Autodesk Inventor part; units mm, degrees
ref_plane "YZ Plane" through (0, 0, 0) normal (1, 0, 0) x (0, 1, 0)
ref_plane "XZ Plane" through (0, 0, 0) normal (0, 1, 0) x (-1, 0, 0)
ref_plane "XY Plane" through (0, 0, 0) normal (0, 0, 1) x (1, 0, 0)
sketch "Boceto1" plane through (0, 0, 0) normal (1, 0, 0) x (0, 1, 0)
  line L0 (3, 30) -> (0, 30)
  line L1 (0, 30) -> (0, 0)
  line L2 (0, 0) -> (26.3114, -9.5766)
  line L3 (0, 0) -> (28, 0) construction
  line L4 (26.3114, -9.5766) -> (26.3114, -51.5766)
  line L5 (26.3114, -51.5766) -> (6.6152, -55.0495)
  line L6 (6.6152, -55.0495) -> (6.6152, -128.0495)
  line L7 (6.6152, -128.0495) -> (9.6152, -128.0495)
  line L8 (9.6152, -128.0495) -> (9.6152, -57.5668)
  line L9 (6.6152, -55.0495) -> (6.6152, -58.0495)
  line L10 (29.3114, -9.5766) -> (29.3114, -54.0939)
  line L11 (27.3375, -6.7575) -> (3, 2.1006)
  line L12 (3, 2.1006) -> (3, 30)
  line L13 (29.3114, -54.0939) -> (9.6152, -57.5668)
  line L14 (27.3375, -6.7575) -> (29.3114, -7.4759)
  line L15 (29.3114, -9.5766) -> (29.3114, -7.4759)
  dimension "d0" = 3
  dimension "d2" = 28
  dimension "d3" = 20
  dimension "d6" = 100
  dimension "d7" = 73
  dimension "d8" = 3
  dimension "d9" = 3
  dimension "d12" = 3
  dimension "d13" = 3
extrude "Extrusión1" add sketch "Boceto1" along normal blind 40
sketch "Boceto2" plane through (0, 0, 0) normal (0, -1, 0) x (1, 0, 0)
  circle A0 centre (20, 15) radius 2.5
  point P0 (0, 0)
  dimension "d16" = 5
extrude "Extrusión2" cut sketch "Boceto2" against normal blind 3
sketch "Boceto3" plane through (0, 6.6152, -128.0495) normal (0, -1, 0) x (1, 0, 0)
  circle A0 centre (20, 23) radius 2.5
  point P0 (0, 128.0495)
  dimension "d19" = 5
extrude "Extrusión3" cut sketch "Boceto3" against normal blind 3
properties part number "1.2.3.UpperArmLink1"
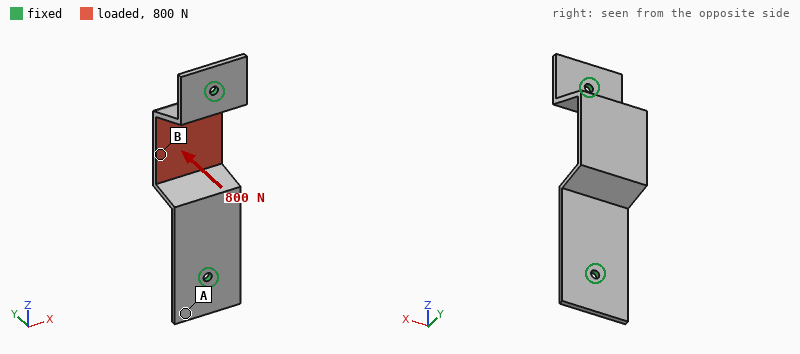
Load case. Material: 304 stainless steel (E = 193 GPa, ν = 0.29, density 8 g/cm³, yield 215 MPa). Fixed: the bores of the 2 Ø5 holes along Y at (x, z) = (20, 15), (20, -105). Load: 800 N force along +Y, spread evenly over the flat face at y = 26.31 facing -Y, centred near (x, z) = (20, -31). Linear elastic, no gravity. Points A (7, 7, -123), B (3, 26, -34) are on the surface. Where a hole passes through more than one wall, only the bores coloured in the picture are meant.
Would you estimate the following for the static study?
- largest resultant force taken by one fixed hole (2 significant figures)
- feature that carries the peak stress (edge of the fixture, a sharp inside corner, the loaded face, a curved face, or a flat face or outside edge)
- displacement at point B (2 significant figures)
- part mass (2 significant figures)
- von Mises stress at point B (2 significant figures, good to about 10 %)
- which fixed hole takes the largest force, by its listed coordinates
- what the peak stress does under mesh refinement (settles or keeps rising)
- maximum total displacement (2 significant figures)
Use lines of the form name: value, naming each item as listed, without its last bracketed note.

largest resultant force taken by one fixed hole: 680 N
feature that carries the peak stress: edge of the fixture
displacement at point B: 0.14 mm
part mass: 180 g
von Mises stress at point B: 28 MPa
which fixed hole takes the largest force, by its listed coordinates: (20, 15)
what the peak stress does under mesh refinement: keeps rising
maximum total displacement: 0.20 mm
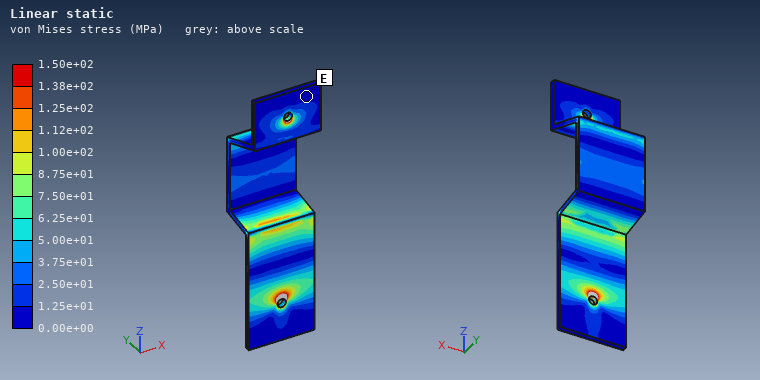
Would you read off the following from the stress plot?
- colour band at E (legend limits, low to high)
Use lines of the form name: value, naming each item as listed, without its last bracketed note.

colour band at E: 0.00e+00 to 1.25e+01 MPa
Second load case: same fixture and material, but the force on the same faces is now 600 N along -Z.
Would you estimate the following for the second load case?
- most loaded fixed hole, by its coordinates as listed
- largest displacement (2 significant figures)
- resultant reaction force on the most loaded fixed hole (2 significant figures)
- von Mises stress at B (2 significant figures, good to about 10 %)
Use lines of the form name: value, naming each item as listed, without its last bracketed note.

most loaded fixed hole, by its coordinates as listed: (20, -105)
largest displacement: 50 µm
resultant reaction force on the most loaded fixed hole: 390 N
von Mises stress at B: 14 MPa
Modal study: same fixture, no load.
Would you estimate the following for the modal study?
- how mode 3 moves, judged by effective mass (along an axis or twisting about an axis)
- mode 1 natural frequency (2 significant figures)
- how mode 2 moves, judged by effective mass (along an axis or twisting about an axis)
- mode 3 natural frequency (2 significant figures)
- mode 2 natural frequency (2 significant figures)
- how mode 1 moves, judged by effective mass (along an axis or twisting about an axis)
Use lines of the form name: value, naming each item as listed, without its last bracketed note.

how mode 3 moves, judged by effective mass: along Z
mode 1 natural frequency: 1000 Hz
how mode 2 moves, judged by effective mass: along X
mode 3 natural frequency: 2400 Hz
mode 2 natural frequency: 1100 Hz
how mode 1 moves, judged by effective mass: along Y
